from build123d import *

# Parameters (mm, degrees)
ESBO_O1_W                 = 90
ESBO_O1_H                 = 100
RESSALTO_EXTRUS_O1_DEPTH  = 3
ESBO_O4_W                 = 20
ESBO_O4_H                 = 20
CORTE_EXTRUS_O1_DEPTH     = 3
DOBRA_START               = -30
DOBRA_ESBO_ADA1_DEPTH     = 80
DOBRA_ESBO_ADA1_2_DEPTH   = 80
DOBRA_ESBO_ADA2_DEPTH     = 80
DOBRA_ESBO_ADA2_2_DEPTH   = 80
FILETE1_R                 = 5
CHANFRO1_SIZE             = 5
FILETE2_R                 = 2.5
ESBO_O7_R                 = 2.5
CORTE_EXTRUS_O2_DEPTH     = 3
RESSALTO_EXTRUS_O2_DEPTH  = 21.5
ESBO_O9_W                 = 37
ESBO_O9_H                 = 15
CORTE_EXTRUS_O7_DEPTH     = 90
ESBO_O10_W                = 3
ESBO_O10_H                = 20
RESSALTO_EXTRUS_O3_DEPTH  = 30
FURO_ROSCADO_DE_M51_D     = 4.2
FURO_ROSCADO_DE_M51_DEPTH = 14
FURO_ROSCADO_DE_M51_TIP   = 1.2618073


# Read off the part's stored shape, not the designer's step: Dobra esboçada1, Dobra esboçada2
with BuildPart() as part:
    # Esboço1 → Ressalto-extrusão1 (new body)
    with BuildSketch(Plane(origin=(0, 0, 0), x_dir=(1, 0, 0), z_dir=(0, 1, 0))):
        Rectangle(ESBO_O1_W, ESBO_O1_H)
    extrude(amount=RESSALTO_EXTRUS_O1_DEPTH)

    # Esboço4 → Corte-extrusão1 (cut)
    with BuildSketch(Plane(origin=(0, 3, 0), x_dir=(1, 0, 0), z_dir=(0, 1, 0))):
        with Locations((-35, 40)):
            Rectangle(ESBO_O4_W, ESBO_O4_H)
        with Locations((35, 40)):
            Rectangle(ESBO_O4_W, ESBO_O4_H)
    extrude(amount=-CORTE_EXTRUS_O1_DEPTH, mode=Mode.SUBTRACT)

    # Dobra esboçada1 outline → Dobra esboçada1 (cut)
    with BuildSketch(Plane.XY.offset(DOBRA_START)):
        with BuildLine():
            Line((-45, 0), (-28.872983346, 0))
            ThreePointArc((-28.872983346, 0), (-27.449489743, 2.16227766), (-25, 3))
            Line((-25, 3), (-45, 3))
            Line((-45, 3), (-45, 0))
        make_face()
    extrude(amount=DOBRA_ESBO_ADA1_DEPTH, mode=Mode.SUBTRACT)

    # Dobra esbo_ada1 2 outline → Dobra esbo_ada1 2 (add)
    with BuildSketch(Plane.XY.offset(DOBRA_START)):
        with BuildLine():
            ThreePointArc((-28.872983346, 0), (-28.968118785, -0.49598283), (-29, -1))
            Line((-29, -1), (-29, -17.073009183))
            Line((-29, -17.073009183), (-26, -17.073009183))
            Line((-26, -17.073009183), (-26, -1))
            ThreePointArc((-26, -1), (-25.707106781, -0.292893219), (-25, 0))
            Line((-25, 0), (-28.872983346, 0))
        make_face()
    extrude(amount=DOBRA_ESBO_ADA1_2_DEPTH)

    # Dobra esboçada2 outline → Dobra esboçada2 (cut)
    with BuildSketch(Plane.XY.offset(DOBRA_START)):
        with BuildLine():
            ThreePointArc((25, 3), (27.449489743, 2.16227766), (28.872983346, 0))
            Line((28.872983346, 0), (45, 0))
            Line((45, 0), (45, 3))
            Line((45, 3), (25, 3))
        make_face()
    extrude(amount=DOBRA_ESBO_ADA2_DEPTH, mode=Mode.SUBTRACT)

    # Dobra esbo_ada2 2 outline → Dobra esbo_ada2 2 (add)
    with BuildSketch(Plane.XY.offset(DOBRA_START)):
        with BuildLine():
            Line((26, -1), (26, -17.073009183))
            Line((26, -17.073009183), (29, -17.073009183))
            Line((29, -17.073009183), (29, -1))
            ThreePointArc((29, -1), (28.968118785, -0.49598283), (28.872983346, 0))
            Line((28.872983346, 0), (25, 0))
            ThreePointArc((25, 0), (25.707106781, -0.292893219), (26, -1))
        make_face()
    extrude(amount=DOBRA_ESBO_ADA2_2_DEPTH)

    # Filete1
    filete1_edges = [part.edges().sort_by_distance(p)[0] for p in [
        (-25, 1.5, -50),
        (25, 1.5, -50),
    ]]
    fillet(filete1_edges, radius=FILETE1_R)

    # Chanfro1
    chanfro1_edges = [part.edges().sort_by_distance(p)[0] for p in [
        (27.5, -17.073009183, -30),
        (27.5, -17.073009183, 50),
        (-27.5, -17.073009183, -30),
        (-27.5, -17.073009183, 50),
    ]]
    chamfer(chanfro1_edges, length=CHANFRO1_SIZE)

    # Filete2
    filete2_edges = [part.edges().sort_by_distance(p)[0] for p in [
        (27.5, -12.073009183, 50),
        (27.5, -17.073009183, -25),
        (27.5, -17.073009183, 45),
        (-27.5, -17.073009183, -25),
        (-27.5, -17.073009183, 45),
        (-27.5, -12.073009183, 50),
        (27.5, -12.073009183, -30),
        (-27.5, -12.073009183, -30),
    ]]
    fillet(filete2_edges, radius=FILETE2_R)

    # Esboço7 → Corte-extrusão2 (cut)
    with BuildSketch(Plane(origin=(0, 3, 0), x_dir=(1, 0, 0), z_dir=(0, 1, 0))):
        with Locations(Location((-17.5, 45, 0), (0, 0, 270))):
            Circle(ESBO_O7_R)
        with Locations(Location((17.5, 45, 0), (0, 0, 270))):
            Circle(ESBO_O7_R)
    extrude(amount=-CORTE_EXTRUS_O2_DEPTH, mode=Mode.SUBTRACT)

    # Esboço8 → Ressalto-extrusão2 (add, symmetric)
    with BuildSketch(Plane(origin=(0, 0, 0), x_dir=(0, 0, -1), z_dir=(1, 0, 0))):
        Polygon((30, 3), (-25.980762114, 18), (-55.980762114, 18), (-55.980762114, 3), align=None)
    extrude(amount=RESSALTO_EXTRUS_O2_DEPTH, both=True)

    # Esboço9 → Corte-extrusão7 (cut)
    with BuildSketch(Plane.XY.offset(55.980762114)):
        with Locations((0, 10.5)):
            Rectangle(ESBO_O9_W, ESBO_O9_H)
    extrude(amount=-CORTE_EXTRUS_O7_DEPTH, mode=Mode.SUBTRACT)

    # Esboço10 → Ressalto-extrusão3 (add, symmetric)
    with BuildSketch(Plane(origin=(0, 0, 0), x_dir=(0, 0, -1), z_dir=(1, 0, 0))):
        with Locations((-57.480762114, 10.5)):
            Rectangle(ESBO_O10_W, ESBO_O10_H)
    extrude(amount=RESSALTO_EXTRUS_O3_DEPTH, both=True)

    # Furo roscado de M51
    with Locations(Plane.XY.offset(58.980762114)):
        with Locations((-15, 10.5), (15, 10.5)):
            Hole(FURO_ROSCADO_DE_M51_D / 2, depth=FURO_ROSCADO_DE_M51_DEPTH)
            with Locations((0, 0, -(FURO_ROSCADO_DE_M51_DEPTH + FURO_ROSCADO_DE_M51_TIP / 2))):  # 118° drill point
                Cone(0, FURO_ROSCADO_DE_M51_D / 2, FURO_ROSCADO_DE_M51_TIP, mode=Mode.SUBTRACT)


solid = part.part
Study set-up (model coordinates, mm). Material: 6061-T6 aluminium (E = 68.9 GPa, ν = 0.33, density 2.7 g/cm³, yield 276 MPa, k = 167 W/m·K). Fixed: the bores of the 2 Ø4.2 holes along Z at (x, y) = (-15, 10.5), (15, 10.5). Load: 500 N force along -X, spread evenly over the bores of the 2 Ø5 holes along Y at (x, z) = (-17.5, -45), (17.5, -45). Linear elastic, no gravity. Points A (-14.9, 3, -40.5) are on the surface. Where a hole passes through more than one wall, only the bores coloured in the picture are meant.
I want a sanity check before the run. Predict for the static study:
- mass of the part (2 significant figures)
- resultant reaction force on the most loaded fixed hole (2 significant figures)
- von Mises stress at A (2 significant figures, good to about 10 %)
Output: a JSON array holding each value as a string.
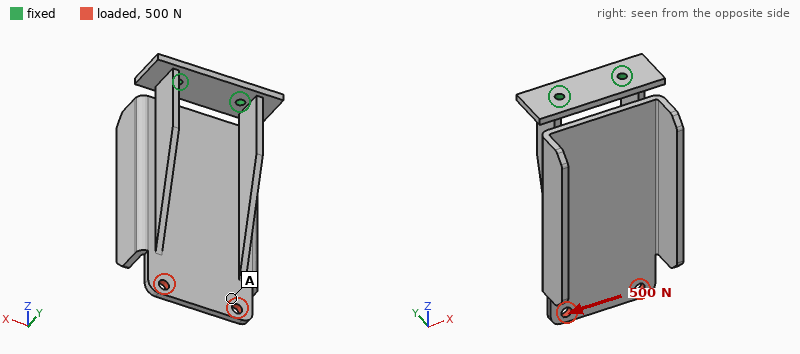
["89 g", "1.3 kN", "16 MPa"]
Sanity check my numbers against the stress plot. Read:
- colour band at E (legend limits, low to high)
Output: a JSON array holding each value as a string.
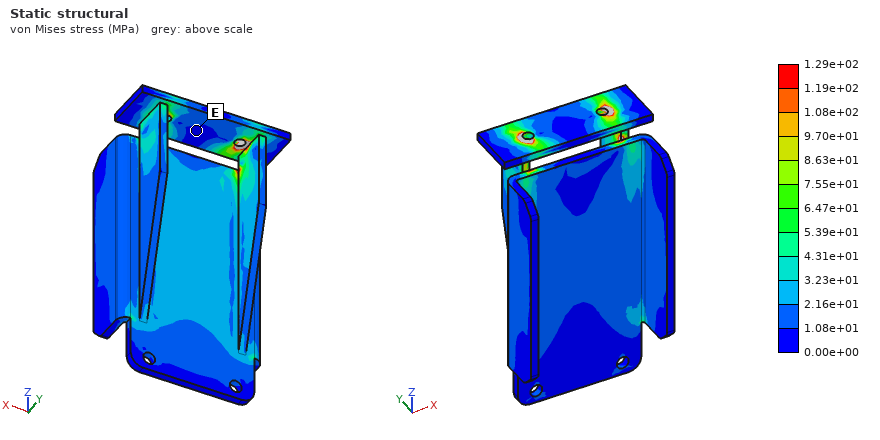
["0.00e+00 to 1.08e+01 MPa"]
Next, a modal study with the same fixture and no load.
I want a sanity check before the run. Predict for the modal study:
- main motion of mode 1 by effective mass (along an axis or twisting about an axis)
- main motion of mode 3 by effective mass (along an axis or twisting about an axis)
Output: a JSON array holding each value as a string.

["along Y", "along X"]
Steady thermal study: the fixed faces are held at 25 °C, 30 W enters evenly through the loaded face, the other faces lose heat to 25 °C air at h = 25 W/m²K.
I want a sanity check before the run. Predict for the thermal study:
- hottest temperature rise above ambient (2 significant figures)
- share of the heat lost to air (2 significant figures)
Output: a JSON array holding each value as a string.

["76 K", "53 %"]
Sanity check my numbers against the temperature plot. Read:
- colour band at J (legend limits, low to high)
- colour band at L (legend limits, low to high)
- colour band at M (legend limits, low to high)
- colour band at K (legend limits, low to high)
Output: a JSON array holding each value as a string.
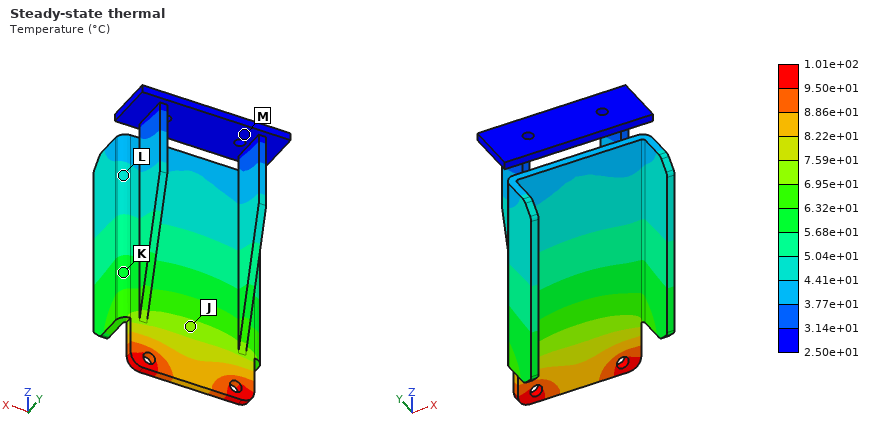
["6.95e+01 to 7.59e+01 °C", "4.41e+01 to 5.04e+01 °C", "2.50e+01 to 3.14e+01 °C", "5.68e+01 to 6.32e+01 °C"]
